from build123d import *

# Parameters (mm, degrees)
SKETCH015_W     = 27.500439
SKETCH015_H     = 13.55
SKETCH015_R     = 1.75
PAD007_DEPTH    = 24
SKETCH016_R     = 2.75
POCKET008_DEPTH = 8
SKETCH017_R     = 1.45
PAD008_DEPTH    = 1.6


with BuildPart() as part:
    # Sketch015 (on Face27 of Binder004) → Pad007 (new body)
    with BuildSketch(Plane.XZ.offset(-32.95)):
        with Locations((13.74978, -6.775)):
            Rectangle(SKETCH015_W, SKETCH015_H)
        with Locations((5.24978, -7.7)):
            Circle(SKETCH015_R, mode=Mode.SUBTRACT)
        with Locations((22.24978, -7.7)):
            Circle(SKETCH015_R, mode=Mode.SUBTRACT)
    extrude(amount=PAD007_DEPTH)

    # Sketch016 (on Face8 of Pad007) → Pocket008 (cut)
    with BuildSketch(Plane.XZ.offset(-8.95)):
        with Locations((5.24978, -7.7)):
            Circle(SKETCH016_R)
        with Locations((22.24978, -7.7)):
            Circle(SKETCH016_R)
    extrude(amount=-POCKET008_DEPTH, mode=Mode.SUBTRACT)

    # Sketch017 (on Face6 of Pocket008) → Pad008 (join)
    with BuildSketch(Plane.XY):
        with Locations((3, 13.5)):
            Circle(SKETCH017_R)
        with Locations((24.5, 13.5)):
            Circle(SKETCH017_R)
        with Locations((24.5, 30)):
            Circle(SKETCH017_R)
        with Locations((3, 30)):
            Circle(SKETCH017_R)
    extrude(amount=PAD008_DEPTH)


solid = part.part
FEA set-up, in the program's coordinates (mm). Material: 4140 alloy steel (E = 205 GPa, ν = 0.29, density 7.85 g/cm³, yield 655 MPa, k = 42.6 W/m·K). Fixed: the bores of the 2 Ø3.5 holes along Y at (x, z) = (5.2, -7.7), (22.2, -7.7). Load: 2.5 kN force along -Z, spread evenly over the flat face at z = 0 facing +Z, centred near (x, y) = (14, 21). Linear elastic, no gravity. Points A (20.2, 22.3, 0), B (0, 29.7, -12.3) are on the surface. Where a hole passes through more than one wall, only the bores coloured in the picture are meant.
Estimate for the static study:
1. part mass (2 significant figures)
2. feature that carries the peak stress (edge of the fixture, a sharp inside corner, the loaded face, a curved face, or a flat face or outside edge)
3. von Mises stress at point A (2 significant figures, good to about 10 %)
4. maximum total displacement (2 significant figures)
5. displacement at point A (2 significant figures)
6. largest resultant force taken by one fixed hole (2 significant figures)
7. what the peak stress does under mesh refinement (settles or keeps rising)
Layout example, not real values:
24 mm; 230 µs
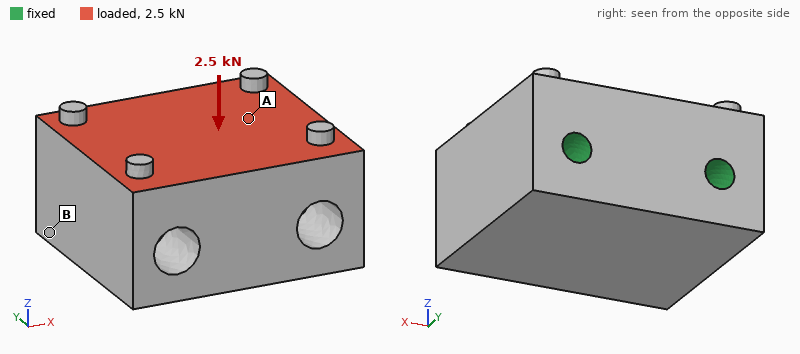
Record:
65 g; edge of the fixture; 8.5 MPa; 1.3 µm; 0.33 µm; 1.3 kN; keeps rising
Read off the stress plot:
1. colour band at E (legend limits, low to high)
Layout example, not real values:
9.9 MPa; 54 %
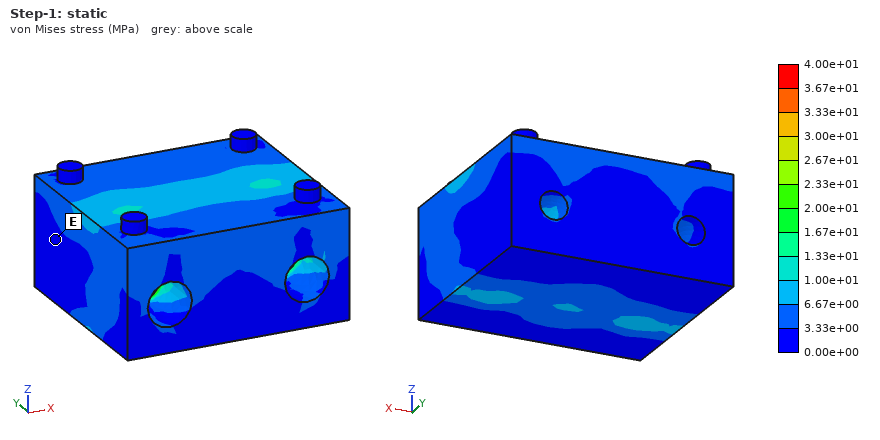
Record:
0.00e+00 to 3.33e+00 MPa
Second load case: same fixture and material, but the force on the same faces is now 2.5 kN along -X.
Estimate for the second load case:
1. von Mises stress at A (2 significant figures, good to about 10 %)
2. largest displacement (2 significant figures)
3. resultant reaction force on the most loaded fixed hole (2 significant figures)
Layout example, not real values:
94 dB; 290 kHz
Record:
9.1 MPa; 1.5 µm; 1.6 kN
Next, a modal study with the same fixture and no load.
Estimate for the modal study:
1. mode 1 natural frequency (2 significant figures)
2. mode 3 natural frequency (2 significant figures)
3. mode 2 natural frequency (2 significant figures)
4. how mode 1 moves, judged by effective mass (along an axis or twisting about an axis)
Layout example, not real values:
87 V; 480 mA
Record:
35 kHz; 50 kHz; 49 kHz; along Z
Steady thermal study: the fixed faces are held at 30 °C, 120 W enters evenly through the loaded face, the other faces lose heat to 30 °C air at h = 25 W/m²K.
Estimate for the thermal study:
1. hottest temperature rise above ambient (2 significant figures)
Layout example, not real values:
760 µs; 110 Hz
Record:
60 K
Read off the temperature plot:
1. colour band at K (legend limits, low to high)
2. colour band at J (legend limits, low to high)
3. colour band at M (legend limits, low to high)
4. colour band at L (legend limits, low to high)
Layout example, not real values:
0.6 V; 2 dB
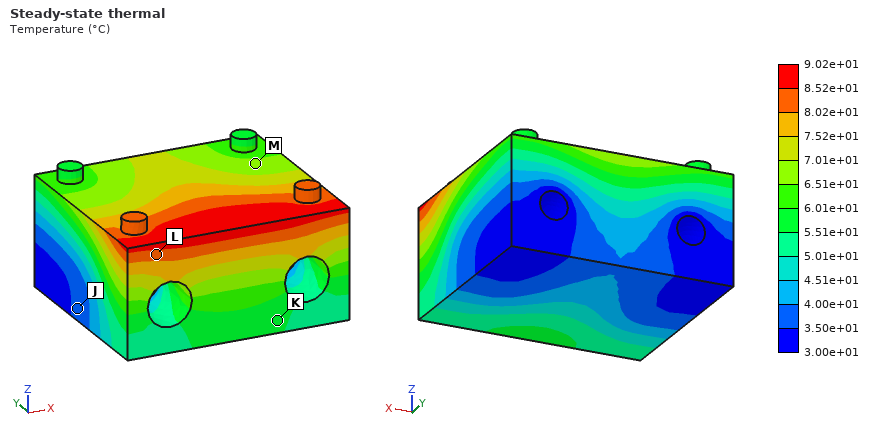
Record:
5.51e+01 to 6.01e+01 °C; 3.50e+01 to 4.00e+01 °C; 6.51e+01 to 7.01e+01 °C; 8.02e+01 to 8.52e+01 °C
